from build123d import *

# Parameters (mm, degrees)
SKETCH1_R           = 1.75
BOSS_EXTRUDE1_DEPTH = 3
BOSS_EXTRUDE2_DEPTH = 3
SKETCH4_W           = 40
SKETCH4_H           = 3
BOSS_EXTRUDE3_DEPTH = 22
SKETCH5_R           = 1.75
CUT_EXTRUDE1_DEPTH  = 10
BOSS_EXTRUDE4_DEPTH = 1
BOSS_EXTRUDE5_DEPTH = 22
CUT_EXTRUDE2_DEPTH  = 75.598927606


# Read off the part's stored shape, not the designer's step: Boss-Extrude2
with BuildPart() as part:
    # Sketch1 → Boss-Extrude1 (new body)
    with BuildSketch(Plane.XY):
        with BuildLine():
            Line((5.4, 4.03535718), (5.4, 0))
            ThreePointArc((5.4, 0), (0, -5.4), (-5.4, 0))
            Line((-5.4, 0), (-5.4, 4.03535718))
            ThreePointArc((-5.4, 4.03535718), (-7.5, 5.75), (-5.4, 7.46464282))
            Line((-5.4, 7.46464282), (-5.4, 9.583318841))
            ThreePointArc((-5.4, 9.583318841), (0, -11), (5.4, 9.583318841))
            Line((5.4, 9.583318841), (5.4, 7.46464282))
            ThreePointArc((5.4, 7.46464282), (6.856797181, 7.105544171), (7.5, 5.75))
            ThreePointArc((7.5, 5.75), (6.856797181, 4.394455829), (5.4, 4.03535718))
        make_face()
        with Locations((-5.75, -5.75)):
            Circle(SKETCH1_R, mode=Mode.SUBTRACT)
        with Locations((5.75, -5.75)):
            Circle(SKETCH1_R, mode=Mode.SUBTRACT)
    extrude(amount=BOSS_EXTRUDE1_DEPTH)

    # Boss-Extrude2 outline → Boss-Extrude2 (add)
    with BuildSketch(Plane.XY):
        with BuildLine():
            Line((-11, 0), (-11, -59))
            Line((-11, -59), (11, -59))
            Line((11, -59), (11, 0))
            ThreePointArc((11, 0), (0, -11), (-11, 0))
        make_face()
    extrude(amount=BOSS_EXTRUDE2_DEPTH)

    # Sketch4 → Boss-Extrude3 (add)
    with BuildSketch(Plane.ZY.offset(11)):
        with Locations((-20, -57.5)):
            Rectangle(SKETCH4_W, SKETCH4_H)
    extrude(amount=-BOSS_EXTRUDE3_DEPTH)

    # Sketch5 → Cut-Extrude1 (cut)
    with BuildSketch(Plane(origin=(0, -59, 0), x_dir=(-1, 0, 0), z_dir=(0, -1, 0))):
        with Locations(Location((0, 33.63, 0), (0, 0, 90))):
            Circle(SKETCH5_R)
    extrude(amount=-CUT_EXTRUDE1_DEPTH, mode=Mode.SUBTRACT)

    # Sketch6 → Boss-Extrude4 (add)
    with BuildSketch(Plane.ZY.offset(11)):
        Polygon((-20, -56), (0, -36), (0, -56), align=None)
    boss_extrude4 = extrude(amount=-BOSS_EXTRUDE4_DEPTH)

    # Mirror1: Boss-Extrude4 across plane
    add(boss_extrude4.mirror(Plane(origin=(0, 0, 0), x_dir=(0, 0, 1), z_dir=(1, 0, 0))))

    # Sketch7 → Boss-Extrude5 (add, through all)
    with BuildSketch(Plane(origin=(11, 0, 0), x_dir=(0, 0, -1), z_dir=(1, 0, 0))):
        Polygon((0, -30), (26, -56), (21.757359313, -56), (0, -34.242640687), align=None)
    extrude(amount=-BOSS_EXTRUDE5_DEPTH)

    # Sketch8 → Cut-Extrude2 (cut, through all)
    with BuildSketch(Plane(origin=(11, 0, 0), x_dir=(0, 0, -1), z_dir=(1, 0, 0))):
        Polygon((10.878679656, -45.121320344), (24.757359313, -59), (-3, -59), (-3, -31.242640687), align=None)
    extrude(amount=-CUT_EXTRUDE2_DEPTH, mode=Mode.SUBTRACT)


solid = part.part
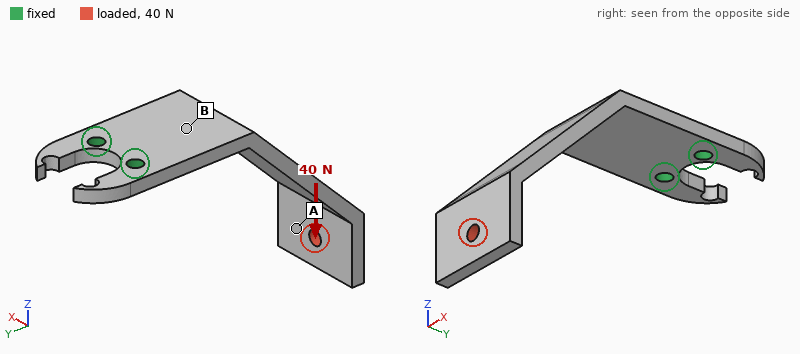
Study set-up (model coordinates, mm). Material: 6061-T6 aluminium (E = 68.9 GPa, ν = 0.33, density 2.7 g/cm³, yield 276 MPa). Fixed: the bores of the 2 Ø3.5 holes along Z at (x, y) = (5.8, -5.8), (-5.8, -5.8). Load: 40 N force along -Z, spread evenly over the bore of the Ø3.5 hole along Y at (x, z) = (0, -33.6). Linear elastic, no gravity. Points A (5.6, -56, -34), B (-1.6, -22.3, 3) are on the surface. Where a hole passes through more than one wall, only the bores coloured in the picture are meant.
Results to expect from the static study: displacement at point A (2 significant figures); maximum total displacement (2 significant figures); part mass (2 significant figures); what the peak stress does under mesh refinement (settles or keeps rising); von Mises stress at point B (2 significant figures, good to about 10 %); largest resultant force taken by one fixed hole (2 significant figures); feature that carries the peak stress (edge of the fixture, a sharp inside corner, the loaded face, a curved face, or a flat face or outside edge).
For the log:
0.74 mm
0.84 mm
15 g
keeps rising
38 MPa
20 N
edge of the fixture
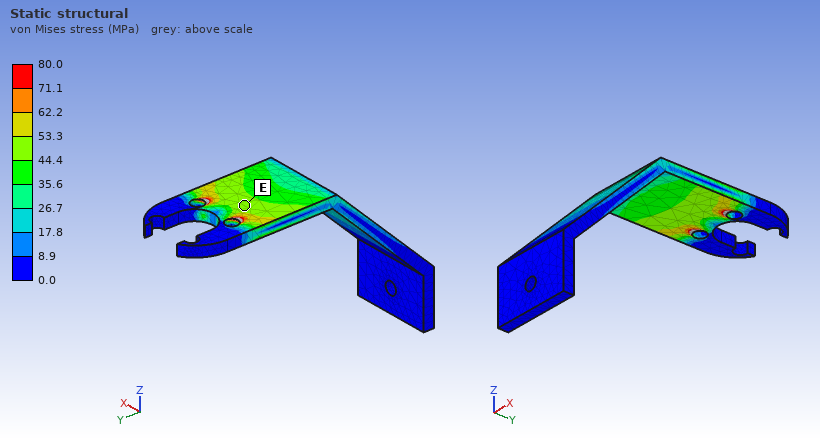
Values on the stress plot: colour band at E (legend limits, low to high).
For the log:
44.4 to 53.3 MPa
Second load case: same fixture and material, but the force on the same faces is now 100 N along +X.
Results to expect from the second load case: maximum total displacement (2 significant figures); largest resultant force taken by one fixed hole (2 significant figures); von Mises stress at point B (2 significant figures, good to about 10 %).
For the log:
0.67 mm
440 N
82 MPa
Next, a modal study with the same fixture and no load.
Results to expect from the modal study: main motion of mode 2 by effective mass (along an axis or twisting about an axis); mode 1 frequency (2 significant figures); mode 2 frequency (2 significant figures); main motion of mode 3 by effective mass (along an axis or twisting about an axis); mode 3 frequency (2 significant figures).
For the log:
along X
460 Hz
1100 Hz
along Z
2200 Hz
